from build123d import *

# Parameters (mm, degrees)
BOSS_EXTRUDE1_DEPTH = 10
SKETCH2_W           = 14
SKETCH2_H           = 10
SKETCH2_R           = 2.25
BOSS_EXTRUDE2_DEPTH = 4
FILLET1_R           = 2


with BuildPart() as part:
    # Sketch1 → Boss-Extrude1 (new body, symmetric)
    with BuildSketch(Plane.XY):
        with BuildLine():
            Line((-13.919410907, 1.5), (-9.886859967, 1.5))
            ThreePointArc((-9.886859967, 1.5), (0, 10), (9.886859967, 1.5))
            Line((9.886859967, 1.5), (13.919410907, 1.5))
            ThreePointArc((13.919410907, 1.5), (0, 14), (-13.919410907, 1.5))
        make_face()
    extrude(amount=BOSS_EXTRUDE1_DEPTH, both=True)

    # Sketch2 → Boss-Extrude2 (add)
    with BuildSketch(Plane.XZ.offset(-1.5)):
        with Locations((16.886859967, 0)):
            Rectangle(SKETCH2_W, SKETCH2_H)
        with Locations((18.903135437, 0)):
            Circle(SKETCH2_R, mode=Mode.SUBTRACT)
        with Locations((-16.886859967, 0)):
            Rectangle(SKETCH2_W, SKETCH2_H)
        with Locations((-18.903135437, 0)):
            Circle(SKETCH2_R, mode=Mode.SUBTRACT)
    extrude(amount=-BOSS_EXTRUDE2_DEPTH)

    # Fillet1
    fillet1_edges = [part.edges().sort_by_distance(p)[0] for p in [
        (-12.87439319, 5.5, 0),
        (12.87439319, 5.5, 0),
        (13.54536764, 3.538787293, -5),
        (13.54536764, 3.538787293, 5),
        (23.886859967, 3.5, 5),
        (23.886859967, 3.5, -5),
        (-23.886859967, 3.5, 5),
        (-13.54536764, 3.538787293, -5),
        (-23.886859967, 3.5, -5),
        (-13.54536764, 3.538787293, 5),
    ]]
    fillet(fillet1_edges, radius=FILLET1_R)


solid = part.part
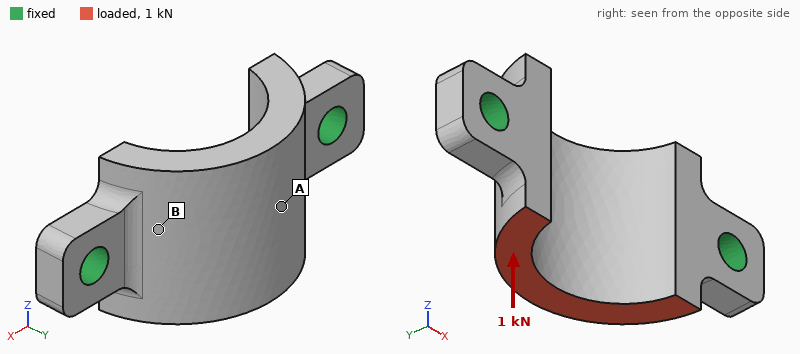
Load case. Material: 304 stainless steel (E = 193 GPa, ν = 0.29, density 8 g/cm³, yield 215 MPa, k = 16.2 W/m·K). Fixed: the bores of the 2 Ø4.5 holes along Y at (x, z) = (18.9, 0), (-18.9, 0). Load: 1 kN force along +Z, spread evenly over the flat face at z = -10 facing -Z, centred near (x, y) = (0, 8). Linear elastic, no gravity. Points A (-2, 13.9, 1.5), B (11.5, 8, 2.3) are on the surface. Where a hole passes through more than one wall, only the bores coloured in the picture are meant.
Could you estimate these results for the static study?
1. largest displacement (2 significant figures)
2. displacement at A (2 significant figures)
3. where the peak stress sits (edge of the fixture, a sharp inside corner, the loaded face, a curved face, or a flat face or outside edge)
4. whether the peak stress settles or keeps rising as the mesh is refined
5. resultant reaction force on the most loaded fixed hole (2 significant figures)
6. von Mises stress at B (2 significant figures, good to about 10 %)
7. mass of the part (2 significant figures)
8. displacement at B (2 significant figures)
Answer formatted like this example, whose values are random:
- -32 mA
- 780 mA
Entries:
- 18 µm
- 14 µm
- edge of the fixture
- keeps rising
- 500 N
- 33 MPa
- 28 g
- 6.9 µm
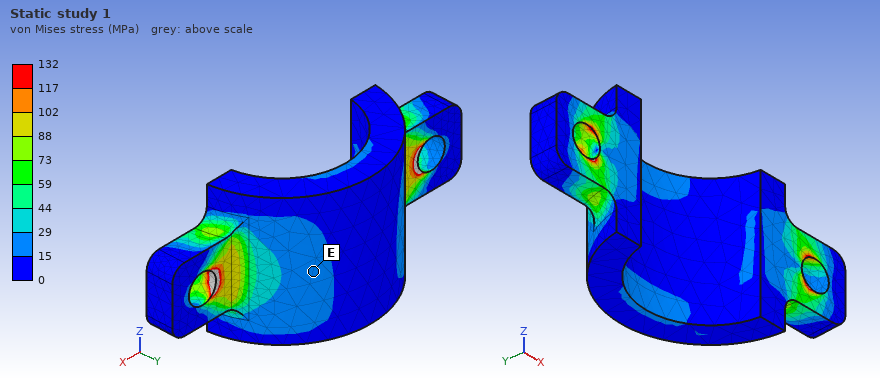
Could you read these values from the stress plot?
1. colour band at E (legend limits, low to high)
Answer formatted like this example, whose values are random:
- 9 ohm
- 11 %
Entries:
- 15 to 29 MPa
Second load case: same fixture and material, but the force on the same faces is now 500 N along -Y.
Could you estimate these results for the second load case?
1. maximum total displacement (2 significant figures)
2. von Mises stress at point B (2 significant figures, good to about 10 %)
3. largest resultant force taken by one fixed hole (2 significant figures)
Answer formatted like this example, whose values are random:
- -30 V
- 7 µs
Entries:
- 16 µm
- 19 MPa
- 330 N
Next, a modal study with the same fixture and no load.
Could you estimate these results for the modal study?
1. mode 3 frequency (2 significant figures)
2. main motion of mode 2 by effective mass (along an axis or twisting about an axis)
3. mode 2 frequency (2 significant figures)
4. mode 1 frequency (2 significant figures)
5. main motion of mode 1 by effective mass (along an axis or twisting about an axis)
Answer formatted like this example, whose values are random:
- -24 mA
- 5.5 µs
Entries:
- 24 kHz
- along Y
- 20 kHz
- 8800 Hz
- along Z
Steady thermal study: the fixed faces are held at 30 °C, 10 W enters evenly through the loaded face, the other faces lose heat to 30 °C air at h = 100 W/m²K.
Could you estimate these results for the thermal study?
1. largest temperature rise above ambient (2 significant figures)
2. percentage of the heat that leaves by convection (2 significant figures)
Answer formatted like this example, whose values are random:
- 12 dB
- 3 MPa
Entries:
- 64 K
- 50 %
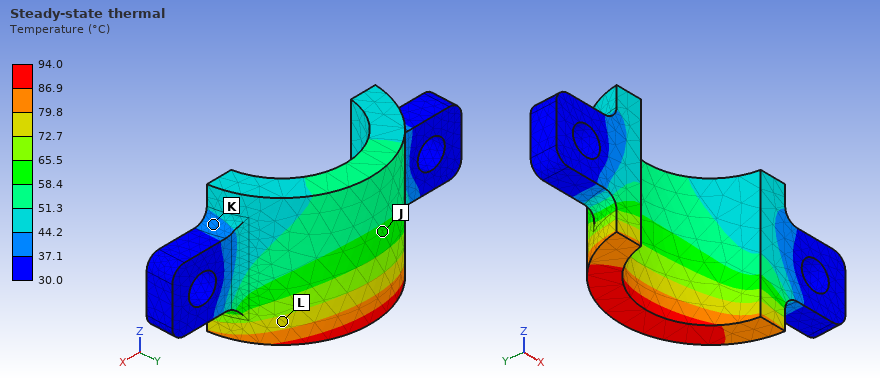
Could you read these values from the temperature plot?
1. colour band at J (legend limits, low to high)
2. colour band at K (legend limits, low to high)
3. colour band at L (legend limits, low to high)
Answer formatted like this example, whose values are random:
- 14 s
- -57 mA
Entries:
- 58.4 to 65.5 °C
- 37.1 to 44.2 °C
- 72.7 to 79.8 °C
